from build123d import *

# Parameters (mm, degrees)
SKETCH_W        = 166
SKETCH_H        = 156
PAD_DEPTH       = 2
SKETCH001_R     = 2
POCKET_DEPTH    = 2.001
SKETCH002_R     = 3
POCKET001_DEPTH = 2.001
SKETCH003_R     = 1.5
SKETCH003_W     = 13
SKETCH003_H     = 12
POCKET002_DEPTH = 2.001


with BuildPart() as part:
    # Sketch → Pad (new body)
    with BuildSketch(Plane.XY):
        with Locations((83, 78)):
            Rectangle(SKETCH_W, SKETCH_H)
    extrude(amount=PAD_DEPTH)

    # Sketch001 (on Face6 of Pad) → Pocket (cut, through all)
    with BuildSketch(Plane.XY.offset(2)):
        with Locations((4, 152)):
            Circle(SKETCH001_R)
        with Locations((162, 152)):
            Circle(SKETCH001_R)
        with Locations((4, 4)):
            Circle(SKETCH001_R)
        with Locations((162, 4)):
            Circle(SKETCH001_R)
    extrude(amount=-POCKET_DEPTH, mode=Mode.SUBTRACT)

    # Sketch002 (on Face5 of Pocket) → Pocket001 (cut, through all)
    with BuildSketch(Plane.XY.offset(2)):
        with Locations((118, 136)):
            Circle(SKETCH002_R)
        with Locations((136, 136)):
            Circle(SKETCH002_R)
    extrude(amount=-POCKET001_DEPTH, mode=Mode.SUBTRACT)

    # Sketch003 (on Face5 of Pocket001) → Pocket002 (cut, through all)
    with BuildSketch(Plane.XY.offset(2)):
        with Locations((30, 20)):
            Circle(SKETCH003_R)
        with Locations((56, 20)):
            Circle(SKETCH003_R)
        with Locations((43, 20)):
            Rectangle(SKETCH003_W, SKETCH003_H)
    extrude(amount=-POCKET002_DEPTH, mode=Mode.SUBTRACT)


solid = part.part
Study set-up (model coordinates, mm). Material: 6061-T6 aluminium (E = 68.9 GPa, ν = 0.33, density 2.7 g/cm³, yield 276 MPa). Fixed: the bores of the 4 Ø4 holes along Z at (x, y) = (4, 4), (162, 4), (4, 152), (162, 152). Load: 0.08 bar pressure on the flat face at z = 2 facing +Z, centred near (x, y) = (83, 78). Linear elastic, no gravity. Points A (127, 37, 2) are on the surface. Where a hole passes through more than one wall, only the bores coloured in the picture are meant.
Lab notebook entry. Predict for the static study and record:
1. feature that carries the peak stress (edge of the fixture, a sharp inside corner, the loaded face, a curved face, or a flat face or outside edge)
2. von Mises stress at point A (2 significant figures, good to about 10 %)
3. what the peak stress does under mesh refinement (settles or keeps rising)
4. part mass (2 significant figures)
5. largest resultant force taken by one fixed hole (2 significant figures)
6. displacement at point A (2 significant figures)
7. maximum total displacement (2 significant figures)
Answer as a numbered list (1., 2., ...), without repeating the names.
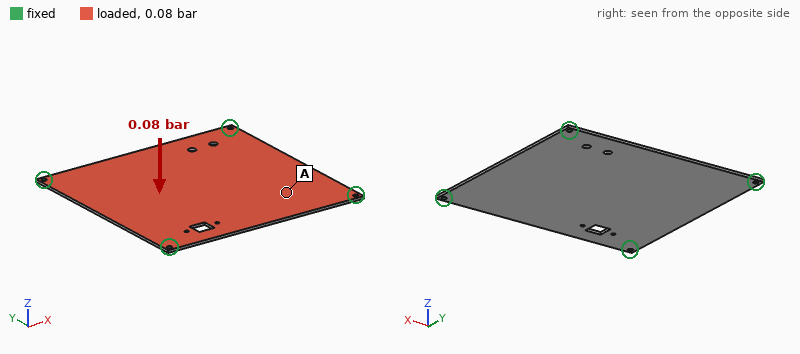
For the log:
1. edge of the fixture
2. 11 MPa
3. keeps rising
4. 140 g
5. 52 N
6. 0.51 mm
7. 0.84 mm
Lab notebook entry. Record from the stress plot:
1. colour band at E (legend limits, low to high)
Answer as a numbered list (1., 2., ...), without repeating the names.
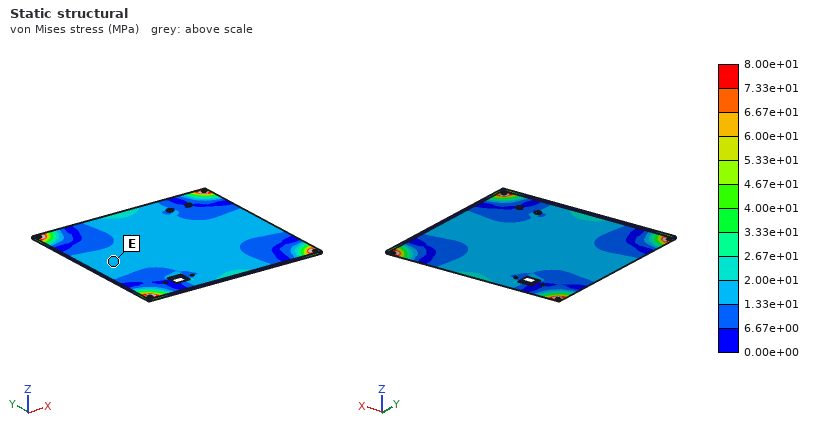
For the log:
1. 1.33e+01 to 2.00e+01 MPa
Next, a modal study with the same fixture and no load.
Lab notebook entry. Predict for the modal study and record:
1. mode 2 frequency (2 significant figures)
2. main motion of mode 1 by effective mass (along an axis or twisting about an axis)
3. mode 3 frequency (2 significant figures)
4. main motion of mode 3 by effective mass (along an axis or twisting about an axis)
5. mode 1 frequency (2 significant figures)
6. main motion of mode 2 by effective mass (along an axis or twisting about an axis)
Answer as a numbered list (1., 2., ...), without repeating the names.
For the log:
1. 450 Hz
2. along Z
3. 480 Hz
4. twisting about Y
5. 250 Hz
6. twisting about X
